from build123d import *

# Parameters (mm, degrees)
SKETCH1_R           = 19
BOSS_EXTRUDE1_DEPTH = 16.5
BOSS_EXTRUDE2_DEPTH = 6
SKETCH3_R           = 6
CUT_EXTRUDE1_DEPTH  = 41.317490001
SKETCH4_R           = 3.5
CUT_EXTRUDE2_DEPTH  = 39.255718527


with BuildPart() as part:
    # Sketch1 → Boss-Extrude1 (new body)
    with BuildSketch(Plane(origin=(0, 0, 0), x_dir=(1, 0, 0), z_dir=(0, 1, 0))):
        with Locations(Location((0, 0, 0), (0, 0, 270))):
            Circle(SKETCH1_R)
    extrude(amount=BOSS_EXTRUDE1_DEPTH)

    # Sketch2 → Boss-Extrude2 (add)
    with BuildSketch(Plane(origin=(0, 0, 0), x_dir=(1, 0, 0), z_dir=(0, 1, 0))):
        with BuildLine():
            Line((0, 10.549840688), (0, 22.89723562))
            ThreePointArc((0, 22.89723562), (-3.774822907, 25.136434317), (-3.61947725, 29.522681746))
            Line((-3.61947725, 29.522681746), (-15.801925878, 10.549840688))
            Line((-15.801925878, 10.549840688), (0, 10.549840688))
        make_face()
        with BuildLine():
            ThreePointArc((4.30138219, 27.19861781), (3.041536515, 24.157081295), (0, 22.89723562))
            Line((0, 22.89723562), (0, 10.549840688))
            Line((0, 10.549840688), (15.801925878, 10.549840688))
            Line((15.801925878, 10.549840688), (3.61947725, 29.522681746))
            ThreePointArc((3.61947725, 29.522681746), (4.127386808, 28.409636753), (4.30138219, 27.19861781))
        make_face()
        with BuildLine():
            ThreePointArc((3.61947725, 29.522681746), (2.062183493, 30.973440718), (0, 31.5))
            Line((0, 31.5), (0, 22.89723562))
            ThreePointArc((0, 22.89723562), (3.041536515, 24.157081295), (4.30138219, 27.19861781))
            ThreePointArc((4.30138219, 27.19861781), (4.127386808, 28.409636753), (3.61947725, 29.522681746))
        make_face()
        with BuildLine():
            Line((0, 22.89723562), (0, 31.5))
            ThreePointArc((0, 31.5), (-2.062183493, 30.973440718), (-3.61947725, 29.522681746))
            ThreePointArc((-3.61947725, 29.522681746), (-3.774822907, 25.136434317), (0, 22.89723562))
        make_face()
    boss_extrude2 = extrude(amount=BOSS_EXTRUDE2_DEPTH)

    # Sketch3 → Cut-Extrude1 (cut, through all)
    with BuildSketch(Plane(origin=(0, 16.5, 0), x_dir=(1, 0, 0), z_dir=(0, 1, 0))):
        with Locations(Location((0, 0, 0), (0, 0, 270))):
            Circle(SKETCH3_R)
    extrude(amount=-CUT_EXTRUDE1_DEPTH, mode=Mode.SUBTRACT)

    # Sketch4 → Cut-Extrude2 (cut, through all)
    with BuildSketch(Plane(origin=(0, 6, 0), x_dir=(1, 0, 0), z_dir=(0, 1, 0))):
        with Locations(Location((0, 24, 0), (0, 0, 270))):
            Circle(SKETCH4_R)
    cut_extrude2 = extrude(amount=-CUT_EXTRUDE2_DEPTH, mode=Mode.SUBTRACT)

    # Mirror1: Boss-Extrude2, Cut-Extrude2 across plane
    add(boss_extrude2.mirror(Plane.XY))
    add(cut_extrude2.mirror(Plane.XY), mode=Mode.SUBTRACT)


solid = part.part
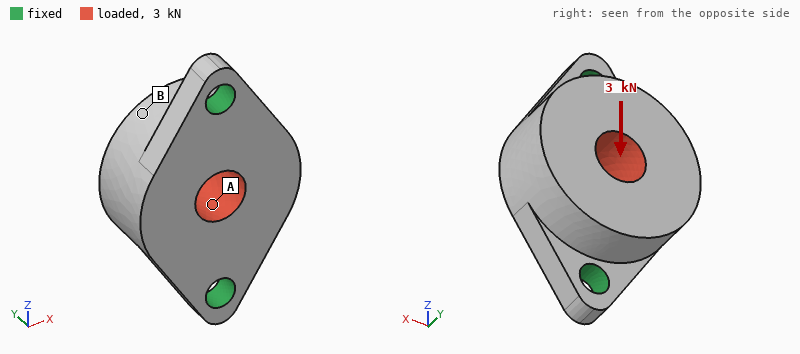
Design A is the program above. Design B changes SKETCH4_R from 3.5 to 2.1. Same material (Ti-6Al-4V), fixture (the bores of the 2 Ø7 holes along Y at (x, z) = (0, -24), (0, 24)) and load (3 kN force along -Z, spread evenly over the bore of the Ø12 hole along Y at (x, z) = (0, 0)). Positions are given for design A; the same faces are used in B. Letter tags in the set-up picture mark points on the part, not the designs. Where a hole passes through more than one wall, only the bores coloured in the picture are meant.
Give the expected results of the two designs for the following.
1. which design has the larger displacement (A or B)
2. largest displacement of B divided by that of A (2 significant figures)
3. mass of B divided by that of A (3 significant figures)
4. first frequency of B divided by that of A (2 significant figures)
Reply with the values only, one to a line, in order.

B
1.3
1.02
0.81
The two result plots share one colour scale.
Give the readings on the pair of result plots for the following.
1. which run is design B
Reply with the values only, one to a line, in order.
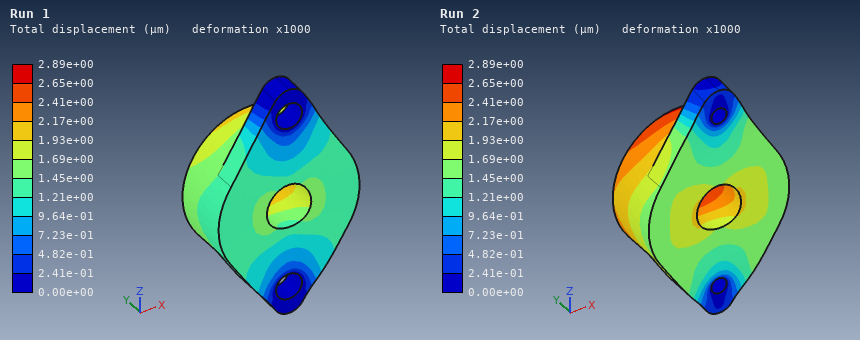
Run 2
